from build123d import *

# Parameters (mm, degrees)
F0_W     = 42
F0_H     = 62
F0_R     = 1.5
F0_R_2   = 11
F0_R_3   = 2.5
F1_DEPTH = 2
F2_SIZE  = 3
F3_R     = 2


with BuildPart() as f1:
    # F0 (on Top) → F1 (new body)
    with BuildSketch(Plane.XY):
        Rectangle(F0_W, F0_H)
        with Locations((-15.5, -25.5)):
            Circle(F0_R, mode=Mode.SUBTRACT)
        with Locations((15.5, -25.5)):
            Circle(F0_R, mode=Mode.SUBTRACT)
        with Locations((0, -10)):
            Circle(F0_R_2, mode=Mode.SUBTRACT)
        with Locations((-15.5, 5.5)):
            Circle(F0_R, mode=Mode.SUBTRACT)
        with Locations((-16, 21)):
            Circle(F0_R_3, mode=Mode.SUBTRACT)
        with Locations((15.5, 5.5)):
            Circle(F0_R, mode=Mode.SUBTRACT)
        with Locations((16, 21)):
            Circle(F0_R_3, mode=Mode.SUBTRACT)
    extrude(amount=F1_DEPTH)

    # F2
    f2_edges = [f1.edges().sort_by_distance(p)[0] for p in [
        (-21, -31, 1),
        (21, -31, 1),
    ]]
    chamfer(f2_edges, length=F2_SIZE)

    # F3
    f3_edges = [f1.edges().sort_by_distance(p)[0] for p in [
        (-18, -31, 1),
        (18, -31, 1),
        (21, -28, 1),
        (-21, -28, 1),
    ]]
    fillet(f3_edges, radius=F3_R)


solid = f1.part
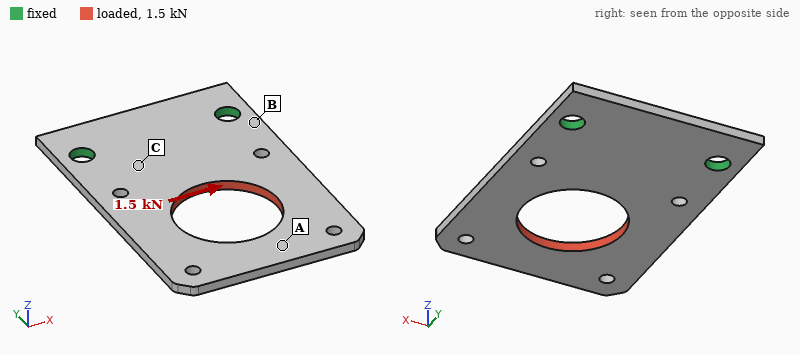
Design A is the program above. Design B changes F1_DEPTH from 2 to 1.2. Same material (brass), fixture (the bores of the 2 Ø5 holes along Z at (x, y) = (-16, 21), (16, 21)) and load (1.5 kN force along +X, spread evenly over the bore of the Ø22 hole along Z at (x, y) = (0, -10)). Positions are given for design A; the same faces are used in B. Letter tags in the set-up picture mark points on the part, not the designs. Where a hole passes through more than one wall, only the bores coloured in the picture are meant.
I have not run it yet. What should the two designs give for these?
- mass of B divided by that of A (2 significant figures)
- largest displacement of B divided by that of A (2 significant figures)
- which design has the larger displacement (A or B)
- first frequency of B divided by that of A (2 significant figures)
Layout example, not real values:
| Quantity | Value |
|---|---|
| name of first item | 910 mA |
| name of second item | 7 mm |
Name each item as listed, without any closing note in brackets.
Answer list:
| Quantity | Value |
|---|---|
| mass of B divided by that of A | 0.60 |
| largest displacement of B divided by that of A | 1.7 |
| which design has the larger displacement | B |
| first frequency of B divided by that of A | 0.61 |
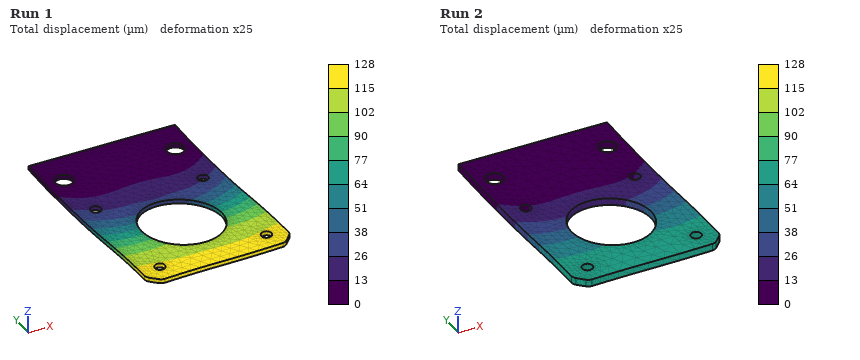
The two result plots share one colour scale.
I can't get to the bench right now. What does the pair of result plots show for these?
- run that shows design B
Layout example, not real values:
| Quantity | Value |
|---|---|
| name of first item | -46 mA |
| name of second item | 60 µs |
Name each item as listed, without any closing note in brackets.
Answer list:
| Quantity | Value |
|---|---|
| run that shows design B | Run 1 |
